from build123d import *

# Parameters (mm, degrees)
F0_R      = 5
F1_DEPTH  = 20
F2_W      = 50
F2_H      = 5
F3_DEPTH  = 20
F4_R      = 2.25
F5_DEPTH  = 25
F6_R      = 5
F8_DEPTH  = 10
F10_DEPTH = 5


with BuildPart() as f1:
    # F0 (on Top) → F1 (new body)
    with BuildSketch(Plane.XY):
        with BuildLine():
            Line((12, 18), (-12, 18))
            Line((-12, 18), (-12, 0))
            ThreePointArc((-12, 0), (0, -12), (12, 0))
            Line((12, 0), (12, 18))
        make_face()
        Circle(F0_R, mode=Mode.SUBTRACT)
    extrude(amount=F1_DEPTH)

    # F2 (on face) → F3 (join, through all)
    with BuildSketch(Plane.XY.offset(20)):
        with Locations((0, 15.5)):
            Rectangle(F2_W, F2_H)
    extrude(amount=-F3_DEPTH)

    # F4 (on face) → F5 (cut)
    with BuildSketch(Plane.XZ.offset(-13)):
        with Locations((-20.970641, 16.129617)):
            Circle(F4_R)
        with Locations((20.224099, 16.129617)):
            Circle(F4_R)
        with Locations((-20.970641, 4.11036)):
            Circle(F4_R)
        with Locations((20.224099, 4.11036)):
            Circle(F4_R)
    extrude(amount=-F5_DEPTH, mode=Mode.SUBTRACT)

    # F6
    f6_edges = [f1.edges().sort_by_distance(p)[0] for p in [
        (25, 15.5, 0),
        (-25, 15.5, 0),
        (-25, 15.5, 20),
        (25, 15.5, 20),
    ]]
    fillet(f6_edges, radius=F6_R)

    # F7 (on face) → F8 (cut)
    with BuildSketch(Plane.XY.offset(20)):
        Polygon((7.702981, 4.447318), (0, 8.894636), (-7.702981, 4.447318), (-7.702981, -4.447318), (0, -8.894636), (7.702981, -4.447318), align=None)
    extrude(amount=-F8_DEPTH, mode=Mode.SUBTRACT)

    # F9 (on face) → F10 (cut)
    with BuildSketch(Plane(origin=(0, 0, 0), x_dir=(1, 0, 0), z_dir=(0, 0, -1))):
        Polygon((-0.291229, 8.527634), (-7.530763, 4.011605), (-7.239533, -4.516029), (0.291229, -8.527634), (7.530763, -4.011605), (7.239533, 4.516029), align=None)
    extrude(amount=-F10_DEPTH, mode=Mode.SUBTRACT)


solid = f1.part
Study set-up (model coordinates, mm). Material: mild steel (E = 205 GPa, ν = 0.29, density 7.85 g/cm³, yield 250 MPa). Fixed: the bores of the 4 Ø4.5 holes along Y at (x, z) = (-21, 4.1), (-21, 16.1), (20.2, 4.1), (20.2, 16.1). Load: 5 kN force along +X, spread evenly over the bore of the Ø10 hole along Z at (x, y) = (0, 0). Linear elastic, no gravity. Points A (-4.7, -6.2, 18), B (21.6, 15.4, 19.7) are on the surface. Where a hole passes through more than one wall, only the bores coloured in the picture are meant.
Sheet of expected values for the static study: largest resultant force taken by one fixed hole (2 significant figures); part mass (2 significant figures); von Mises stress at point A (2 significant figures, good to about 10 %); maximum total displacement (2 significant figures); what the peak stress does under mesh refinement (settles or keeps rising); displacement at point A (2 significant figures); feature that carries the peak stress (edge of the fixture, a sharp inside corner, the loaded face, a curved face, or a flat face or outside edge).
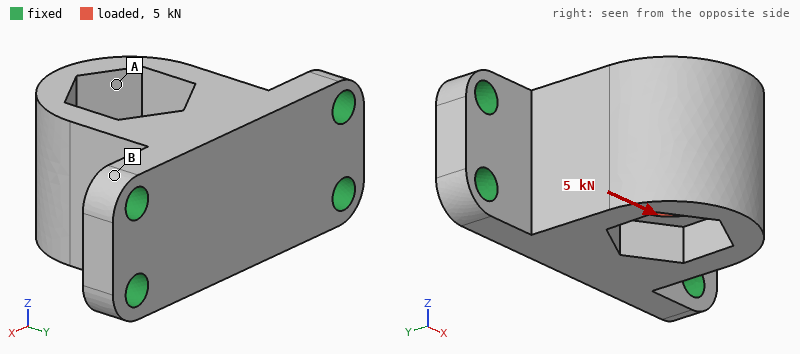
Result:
1.9 kN
94 g
33 MPa
25 µm
keeps rising
21 µm
edge of the fixture
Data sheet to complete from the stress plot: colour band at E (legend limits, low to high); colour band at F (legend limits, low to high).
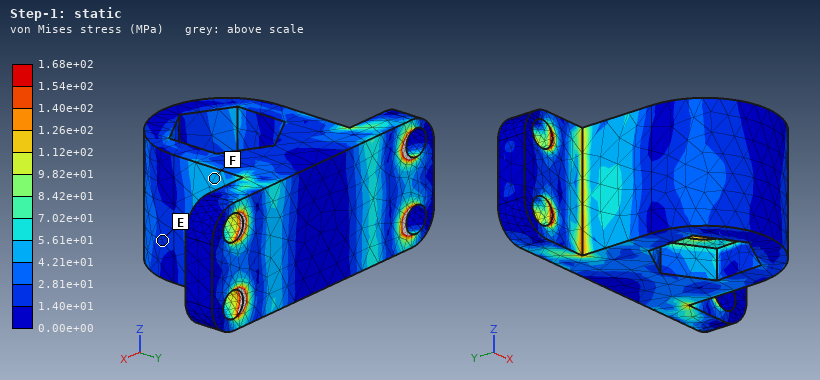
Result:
1.40e+01 to 2.81e+01 MPa
4.21e+01 to 5.61e+01 MPa
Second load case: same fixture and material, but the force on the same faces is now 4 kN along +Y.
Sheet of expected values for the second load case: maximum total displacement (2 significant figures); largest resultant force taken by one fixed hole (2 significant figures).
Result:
15 µm
1.5 kN
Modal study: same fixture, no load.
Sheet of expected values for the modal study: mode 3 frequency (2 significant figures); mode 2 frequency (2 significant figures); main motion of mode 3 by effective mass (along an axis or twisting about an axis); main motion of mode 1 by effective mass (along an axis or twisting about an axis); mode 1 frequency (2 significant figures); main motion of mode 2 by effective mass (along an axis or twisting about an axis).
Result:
13 kHz
12 kHz
along Y
along Z
6400 Hz
along X
